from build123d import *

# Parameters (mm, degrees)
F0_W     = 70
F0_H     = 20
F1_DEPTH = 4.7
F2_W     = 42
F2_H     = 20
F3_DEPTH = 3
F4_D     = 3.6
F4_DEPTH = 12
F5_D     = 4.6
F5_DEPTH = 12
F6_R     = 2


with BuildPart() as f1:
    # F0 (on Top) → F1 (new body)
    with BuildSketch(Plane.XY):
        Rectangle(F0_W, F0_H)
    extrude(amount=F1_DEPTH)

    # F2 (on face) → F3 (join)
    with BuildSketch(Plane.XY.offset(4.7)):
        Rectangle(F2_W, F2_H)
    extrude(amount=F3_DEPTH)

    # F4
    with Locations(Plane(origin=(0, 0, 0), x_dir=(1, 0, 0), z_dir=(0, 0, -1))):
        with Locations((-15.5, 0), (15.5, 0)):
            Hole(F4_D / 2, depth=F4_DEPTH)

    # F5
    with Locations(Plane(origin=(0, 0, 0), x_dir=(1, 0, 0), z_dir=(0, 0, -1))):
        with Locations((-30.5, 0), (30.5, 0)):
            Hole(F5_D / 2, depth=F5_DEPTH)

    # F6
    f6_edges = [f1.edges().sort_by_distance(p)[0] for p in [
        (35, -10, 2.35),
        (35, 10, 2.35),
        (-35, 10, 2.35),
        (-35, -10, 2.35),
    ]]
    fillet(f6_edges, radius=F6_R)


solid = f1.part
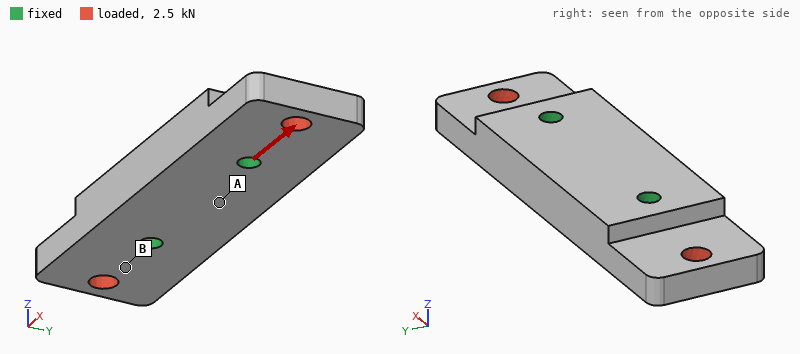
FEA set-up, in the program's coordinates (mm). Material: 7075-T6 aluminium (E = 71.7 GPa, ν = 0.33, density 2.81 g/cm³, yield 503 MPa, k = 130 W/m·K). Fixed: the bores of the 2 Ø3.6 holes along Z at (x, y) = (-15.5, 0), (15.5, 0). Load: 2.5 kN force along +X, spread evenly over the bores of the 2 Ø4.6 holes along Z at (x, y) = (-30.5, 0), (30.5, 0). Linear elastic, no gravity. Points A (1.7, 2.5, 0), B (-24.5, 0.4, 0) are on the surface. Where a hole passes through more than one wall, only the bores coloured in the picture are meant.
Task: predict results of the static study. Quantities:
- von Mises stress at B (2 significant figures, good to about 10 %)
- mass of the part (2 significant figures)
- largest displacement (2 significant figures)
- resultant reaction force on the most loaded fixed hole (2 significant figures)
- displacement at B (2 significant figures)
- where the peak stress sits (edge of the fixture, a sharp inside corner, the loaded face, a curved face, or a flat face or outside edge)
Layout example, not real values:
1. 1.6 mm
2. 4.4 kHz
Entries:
1. 23 MPa
2. 25 g
3. 7.9 µm
4. 1.3 kN
5. 3.1 µm
6. the loaded face
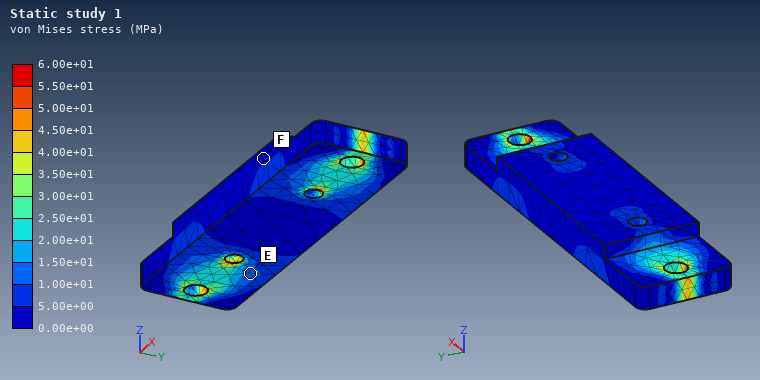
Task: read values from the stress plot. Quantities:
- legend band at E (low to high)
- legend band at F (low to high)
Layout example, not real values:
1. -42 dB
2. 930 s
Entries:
1. 1.00e+01 to 1.50e+01 MPa
2. 0.00e+00 to 5.00e+00 MPa
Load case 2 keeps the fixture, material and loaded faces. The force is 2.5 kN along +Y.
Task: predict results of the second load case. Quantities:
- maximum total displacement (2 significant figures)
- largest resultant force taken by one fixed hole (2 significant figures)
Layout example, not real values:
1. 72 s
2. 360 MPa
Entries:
1. 31 µm
2. 1.3 kN
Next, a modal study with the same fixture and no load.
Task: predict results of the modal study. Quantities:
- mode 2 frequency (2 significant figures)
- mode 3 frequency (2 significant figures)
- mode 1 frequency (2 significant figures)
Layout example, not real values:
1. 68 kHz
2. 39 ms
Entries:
1. 13 kHz
2. 21 kHz
3. 13 kHz
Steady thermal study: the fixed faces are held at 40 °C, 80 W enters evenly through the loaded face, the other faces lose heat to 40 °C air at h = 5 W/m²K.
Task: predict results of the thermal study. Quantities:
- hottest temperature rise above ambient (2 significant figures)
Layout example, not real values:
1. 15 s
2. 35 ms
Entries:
1. 63 K
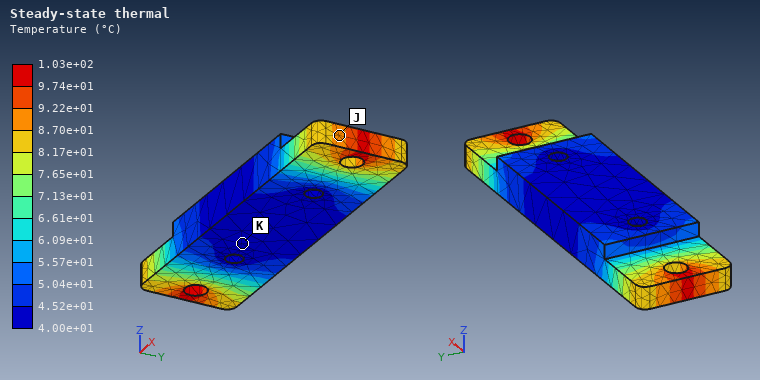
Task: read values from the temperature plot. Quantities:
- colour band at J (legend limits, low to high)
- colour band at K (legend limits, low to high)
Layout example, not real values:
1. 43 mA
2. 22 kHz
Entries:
1. 8.70e+01 to 9.22e+01 °C
2. 4.00e+01 to 4.52e+01 °C
